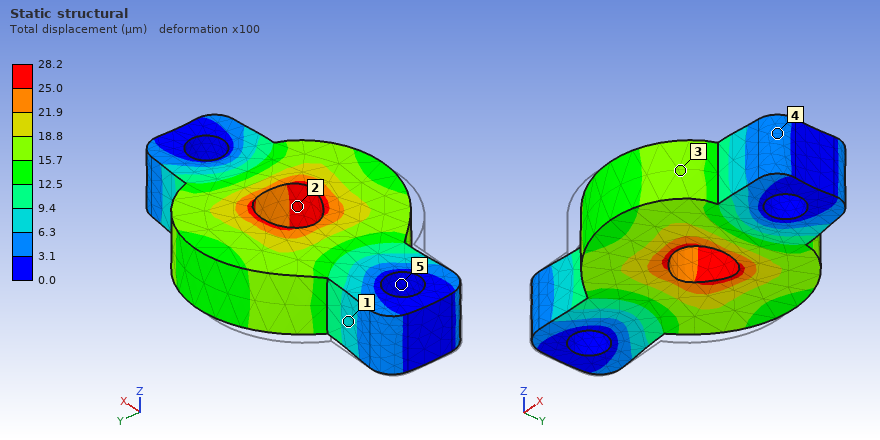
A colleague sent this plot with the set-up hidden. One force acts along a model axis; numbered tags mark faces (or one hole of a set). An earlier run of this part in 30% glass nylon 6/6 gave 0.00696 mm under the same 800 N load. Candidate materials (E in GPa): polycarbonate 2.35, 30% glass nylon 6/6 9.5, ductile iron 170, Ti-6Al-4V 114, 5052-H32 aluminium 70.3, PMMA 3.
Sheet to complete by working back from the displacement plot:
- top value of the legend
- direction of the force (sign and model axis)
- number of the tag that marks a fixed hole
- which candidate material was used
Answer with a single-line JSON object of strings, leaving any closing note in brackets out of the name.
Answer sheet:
{"top value of the legend": "28.2 µm", "direction of the force": "+X", "number of the tag that marks a fixed hole": "5", "which candidate material was used": "polycarbonate"}
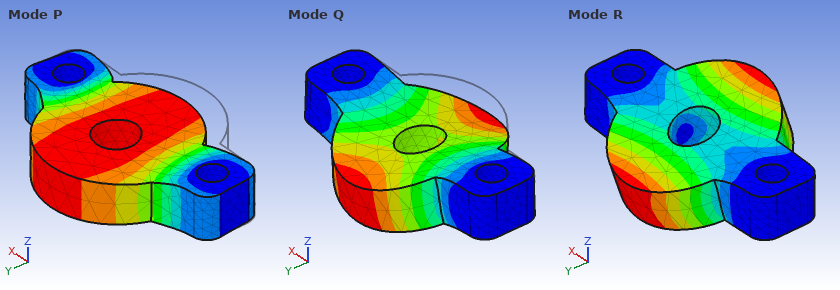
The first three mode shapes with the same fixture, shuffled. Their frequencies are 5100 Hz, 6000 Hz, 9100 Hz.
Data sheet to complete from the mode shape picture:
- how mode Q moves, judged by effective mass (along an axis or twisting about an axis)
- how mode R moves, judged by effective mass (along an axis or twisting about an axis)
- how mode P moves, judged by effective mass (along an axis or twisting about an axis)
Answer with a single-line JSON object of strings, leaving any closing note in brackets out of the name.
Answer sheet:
{"how mode Q moves, judged by effective mass": "along Z", "how mode R moves, judged by effective mass": "twisting about X", "how mode P moves, judged by effective mass": "along Y"}
